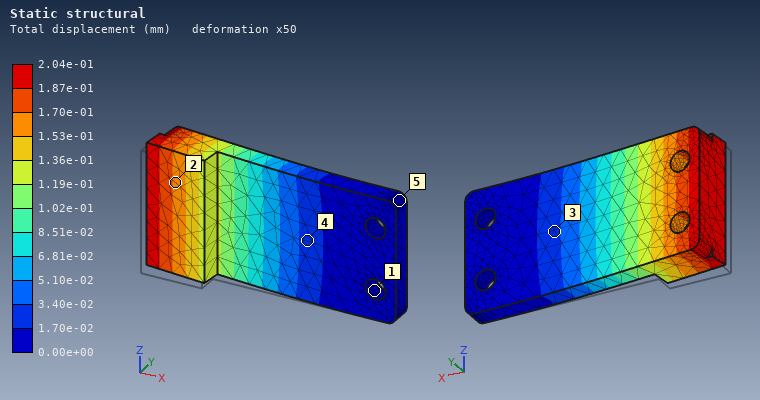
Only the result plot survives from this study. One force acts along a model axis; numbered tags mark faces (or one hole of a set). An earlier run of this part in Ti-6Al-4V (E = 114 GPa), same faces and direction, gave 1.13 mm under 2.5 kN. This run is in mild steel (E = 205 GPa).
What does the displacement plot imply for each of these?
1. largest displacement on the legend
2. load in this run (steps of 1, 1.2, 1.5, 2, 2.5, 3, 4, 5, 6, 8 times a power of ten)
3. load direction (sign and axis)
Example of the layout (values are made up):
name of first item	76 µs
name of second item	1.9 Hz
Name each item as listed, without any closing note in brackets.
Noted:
largest displacement on the legend	2.04e-01 mm
load in this run	800 N
load direction	+Y
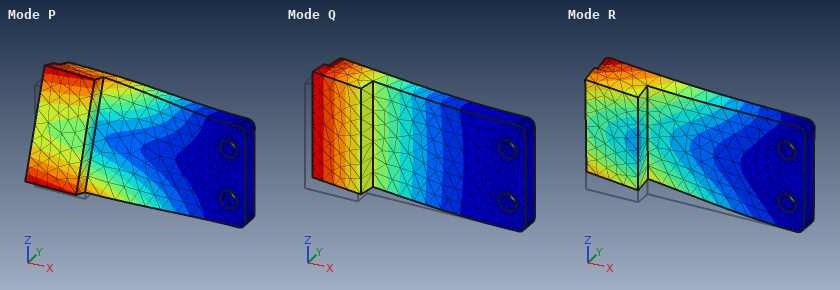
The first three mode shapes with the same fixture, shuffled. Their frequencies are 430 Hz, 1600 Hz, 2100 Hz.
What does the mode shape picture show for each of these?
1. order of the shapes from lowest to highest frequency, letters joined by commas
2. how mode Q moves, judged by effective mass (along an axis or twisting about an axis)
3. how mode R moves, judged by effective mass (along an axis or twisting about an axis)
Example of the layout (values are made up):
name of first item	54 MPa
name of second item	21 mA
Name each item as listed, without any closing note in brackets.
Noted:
order of the shapes from lowest to highest frequency, letters joined by commas	Q, P, R
how mode Q moves, judged by effective mass	along Y
how mode R moves, judged by effective mass	along Z
